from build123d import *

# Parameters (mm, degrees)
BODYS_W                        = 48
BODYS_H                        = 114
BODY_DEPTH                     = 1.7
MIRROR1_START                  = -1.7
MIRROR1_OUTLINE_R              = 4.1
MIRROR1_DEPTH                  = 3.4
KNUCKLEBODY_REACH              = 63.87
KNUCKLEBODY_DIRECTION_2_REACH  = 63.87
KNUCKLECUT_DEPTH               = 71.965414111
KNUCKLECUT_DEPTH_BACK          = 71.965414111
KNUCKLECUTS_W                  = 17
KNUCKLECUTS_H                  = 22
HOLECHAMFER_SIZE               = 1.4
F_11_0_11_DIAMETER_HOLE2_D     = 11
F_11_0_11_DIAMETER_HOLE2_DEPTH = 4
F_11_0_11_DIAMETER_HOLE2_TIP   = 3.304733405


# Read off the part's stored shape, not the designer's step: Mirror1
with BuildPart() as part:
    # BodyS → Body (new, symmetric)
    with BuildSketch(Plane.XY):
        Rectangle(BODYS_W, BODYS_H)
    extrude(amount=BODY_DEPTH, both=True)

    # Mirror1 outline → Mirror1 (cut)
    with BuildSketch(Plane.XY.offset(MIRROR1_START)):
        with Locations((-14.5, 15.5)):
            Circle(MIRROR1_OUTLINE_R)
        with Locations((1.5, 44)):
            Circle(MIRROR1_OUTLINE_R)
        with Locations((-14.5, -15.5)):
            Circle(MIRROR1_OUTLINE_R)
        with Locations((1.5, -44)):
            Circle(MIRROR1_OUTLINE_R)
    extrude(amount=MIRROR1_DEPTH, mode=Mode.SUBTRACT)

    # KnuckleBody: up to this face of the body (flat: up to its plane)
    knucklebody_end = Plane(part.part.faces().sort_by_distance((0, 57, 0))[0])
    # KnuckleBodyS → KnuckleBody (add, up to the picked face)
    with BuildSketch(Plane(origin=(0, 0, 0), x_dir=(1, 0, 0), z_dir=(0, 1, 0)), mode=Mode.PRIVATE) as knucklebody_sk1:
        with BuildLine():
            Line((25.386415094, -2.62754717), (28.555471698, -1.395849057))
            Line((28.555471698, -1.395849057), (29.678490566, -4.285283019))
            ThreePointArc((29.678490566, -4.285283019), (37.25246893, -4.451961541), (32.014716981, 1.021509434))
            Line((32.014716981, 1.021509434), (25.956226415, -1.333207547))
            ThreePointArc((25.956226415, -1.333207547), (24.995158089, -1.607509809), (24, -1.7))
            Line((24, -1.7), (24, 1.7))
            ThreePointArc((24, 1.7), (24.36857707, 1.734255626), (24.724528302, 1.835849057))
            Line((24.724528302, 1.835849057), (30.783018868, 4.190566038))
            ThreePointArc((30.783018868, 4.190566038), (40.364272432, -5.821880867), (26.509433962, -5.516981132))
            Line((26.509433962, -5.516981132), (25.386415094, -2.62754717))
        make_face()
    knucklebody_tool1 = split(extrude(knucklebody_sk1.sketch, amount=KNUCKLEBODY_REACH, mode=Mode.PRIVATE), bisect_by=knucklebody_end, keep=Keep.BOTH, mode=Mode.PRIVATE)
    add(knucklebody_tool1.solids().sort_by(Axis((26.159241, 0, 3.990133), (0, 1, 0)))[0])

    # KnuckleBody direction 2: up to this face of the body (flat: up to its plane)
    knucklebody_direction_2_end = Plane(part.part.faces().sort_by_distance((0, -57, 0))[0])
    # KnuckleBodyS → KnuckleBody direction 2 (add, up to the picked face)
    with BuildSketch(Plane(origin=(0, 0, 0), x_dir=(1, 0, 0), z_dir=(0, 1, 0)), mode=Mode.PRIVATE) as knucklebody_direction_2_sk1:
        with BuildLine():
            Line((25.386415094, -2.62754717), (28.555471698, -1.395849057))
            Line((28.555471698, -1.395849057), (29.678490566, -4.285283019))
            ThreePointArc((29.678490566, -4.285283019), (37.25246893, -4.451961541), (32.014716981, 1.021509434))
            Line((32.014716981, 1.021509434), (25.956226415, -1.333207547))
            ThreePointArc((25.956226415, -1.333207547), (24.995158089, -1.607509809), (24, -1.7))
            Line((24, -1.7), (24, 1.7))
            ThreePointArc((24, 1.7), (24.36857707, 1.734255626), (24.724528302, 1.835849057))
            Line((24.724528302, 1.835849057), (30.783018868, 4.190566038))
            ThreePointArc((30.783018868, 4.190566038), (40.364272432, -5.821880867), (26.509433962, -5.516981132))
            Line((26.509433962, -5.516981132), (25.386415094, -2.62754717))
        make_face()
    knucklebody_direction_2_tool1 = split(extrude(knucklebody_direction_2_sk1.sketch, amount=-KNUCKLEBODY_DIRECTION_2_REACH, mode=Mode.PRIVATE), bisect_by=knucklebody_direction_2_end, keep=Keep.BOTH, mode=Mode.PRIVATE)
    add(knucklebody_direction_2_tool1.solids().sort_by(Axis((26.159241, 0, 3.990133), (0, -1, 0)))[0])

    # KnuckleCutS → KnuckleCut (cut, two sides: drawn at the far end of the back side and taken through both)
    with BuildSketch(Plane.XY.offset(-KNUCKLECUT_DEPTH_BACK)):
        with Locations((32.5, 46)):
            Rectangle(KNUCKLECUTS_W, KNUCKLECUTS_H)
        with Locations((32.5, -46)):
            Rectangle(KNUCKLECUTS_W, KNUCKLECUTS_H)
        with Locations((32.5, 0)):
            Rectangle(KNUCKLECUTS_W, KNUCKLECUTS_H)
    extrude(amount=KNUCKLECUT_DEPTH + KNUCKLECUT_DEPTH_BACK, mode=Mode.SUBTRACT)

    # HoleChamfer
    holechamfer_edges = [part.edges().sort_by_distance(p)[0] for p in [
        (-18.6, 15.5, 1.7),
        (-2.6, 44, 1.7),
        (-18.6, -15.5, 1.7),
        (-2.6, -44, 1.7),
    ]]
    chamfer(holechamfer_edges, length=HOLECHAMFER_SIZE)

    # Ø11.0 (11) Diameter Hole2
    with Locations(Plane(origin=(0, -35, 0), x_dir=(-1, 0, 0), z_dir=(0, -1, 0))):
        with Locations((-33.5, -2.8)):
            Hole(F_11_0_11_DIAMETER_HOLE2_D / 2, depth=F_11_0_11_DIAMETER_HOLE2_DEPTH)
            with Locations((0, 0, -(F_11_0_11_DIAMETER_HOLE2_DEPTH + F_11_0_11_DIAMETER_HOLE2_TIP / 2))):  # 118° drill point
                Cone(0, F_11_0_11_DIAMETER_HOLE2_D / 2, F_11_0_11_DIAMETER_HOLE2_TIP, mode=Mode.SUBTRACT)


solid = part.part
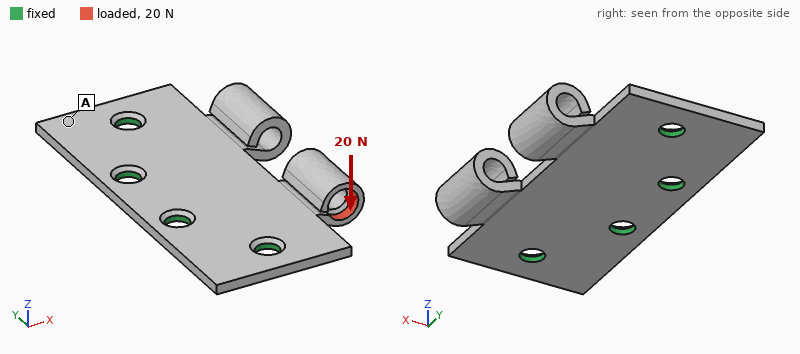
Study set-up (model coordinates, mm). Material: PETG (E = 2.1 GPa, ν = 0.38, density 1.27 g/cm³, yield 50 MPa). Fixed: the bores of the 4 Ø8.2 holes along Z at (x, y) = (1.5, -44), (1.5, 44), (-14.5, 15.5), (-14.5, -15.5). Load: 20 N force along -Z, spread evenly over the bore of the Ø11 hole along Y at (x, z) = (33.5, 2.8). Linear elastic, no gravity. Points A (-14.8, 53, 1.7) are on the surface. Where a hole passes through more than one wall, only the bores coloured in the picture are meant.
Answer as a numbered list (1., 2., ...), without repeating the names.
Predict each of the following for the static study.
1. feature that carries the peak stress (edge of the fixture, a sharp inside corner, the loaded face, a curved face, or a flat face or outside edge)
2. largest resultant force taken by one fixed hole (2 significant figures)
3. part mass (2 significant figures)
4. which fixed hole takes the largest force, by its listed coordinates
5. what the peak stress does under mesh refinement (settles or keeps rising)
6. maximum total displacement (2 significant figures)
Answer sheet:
1. edge of the fixture
2. 21 N
3. 30 g
4. (1.5, -44)
5. keeps rising
6. 1.3 mm
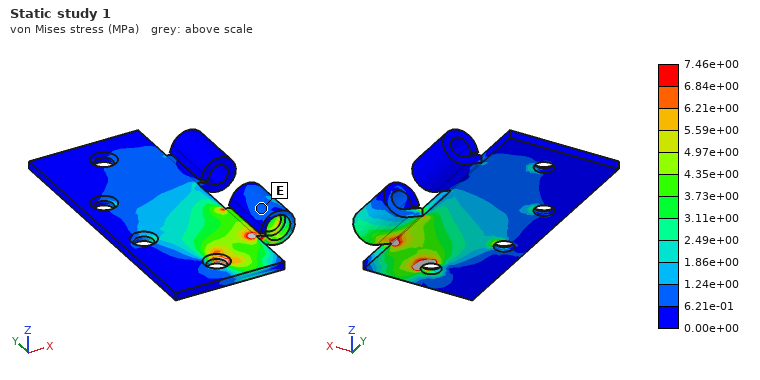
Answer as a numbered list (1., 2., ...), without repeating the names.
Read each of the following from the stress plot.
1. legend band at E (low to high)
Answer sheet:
1. 6.21e-01 to 1.24e+00 MPa
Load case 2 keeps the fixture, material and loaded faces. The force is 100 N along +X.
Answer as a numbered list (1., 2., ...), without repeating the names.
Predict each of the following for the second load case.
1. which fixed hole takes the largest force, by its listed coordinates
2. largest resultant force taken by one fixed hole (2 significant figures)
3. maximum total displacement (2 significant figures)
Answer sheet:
1. (1.5, -44)
2. 64 N
3. 1.4 mm
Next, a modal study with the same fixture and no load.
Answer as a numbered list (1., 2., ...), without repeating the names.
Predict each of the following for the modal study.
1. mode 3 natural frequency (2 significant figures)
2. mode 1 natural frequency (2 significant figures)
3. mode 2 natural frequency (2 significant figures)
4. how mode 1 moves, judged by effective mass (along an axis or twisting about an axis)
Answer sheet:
1. 840 Hz
2. 310 Hz
3. 430 Hz
4. along Z
